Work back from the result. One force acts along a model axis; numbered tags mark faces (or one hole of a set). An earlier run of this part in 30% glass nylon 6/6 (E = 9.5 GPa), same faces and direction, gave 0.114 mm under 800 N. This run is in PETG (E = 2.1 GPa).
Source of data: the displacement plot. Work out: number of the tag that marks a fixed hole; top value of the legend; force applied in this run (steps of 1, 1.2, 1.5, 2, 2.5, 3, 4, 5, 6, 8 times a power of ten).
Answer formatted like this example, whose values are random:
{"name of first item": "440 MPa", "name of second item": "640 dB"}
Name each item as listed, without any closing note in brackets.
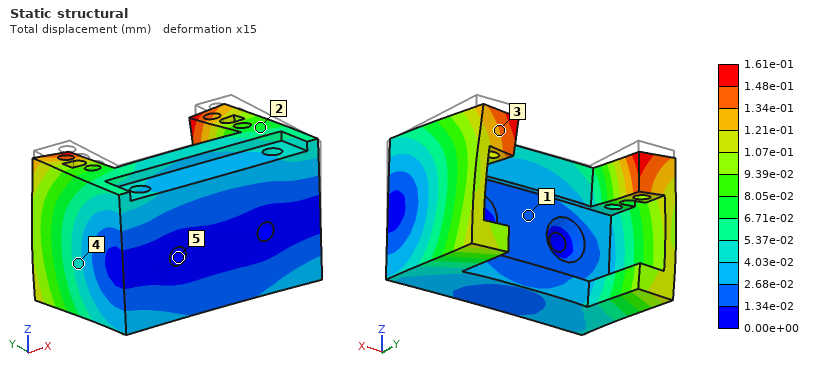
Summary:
{"number of the tag that marks a fixed hole": "5", "top value of the legend": "1.61e-01 mm", "force applied in this run": "250 N"}
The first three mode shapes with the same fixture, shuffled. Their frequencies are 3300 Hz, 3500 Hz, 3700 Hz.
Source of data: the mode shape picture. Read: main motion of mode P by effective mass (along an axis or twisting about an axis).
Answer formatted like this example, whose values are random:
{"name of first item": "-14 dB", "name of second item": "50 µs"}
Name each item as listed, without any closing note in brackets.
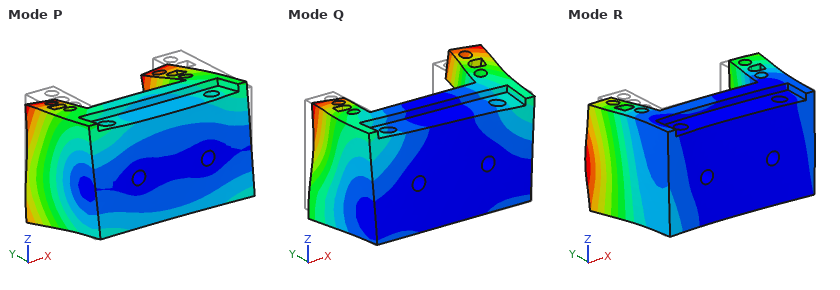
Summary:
{"main motion of mode P by effective mass": "along Z"}
